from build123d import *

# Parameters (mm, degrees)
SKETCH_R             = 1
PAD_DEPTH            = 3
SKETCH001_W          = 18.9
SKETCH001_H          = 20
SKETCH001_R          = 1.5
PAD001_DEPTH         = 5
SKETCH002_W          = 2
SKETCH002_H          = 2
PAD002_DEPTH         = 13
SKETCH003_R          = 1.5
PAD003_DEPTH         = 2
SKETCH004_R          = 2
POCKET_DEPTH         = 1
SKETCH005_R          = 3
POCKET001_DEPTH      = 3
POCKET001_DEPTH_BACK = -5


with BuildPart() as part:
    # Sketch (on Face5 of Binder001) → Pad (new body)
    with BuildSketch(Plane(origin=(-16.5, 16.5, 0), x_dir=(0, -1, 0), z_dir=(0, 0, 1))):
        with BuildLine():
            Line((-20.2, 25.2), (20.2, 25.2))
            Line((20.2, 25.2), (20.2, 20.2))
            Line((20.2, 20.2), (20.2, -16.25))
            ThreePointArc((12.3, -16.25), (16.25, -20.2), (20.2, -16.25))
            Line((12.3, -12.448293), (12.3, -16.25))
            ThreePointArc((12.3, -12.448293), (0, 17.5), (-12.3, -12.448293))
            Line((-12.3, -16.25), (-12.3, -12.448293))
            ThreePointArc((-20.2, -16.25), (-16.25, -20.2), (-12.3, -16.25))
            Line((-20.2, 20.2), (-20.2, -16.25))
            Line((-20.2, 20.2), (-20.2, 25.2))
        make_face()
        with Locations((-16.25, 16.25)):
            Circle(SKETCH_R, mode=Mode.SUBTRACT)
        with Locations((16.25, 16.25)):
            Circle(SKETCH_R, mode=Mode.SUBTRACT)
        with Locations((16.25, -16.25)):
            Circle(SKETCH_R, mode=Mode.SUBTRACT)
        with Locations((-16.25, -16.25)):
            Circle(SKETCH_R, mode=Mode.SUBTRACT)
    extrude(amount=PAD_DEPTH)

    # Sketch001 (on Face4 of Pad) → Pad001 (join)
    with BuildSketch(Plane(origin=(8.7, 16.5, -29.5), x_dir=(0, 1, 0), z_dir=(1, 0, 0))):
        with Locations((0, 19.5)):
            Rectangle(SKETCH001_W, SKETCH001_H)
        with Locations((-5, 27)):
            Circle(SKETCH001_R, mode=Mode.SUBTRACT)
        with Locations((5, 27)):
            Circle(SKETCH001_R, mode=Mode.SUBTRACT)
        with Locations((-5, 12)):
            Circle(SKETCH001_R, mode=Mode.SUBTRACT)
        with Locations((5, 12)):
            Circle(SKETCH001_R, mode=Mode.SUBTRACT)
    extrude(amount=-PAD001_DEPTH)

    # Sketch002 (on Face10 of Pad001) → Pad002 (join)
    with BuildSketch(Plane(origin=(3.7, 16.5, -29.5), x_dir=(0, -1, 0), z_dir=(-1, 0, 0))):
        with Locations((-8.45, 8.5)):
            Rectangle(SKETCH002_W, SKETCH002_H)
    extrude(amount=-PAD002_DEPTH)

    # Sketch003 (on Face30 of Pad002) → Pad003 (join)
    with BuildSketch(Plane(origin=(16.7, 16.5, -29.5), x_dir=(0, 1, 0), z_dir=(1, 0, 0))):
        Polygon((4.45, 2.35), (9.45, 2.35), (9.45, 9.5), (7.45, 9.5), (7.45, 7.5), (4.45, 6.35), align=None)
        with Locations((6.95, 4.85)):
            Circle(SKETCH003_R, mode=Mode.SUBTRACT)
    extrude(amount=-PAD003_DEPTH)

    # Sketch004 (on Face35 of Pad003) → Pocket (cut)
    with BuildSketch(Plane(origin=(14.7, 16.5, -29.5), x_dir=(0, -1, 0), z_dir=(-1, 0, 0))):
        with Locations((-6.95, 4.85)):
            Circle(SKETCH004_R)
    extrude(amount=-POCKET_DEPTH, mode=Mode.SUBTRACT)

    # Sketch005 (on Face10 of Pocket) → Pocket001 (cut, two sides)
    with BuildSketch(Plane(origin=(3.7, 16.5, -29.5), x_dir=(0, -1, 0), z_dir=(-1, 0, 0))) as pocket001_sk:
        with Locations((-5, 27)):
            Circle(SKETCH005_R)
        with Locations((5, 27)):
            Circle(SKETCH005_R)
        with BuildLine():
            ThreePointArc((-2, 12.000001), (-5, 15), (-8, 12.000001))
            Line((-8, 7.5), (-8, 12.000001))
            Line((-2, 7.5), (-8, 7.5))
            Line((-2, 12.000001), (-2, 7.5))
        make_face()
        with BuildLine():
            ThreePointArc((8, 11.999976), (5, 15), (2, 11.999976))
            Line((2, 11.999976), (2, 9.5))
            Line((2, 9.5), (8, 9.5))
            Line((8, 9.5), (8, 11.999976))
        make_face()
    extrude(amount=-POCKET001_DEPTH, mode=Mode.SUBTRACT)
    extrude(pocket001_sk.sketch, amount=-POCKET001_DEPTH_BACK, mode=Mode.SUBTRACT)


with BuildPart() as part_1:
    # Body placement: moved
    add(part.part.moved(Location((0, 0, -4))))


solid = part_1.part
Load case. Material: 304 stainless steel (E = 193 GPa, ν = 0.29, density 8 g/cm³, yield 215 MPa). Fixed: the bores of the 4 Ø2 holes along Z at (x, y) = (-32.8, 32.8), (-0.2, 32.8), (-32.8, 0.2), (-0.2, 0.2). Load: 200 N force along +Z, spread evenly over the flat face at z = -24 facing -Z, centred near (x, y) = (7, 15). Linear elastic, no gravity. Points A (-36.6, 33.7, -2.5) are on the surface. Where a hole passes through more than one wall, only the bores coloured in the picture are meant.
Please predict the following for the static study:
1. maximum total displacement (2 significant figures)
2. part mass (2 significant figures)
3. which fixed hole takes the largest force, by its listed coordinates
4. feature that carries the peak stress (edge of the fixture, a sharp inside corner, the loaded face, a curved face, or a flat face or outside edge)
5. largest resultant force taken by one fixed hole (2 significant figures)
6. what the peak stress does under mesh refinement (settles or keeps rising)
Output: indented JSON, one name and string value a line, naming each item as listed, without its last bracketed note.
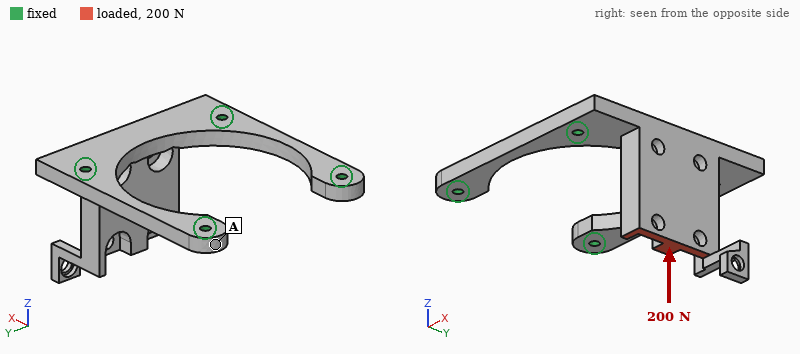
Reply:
{
  "maximum total displacement": "29 µm",
  "part mass": "30 g",
  "which fixed hole takes the largest force, by its listed coordinates": "(-0.2, 0.2)",
  "feature that carries the peak stress": "edge of the fixture",
  "largest resultant force taken by one fixed hole": "110 N",
  "what the peak stress does under mesh refinement": "keeps rising"
}
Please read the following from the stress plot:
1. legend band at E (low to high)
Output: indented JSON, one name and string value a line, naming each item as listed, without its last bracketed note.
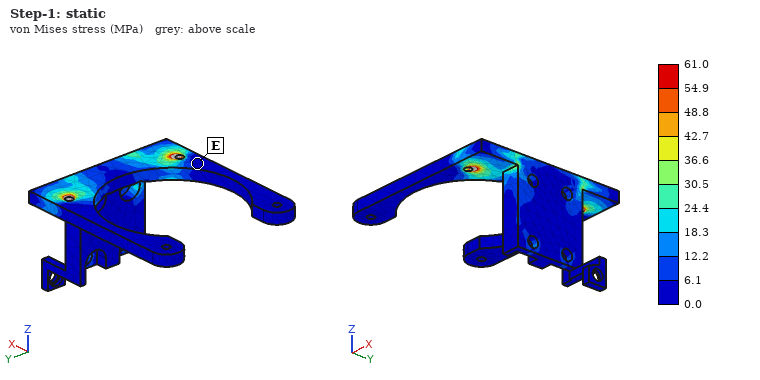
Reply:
{
  "legend band at E": "0.0 to 6.1 MPa"
}
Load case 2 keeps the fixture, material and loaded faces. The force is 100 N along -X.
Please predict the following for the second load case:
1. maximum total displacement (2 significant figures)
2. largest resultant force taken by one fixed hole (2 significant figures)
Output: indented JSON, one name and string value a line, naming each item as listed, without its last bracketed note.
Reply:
{
  "maximum total displacement": "88 µm",
  "largest resultant force taken by one fixed hole": "75 N"
}
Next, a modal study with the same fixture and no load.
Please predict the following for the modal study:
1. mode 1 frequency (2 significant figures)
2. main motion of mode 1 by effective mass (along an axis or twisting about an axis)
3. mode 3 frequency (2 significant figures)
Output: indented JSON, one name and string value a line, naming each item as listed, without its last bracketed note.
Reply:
{
  "mode 1 frequency": "2900 Hz",
  "main motion of mode 1 by effective mass": "along X",
  "mode 3 frequency": "7600 Hz"
}
